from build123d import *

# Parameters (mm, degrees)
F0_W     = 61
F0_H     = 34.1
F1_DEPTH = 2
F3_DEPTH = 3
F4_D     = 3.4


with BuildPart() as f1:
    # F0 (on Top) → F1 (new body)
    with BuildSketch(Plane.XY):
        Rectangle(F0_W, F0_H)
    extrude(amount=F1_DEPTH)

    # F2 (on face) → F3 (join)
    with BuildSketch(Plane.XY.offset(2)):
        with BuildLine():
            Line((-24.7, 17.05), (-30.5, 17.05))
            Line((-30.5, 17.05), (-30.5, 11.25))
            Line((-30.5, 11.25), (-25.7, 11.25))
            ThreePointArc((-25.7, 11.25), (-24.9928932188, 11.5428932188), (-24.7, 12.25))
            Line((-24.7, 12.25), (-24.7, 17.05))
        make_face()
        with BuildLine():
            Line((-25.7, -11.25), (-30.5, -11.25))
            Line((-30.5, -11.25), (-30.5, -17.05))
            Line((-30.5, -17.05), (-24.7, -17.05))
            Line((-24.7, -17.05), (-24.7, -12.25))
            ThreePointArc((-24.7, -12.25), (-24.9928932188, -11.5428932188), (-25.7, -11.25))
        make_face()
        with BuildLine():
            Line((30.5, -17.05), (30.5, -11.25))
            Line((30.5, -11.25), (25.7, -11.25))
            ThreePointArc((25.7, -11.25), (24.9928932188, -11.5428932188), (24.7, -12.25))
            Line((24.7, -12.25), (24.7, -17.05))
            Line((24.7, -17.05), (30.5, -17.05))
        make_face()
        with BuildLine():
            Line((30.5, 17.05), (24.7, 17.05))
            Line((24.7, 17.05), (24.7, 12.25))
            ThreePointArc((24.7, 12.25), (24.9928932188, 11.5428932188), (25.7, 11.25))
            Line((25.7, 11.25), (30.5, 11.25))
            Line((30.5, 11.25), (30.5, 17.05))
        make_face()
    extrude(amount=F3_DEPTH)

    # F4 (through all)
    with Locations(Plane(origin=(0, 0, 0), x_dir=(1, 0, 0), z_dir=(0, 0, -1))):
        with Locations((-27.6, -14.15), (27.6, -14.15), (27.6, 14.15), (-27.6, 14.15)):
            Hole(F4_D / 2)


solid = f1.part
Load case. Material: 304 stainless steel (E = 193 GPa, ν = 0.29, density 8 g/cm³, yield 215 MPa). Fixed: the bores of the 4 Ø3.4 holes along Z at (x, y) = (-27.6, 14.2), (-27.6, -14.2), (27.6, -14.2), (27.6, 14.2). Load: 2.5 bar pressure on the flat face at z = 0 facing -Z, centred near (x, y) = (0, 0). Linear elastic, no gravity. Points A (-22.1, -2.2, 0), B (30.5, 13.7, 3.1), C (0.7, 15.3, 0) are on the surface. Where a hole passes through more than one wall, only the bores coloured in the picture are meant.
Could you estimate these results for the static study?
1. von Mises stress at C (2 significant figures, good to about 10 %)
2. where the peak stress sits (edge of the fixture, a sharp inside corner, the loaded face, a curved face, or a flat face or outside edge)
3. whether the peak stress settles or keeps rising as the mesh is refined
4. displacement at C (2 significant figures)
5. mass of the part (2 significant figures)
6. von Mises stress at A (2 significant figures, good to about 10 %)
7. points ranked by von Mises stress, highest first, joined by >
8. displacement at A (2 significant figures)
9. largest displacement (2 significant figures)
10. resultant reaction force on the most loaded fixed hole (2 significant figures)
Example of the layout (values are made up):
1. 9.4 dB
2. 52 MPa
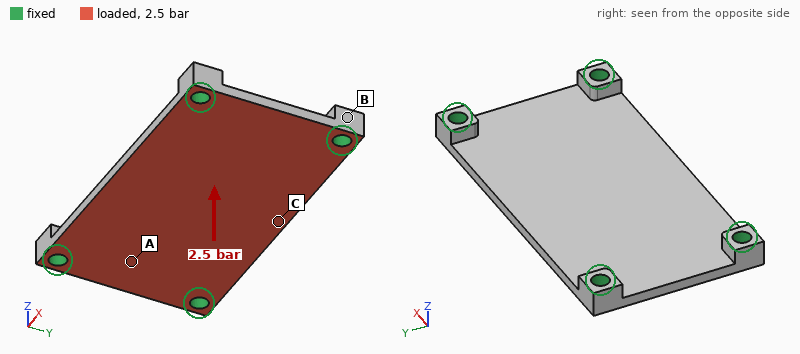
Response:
1. 51 MPa
2. a sharp inside corner
3. keeps rising
4. 46 µm
5. 35 g
6. 28 MPa
7. C > A > B
8. 11 µm
9. 47 µm
10. 130 N
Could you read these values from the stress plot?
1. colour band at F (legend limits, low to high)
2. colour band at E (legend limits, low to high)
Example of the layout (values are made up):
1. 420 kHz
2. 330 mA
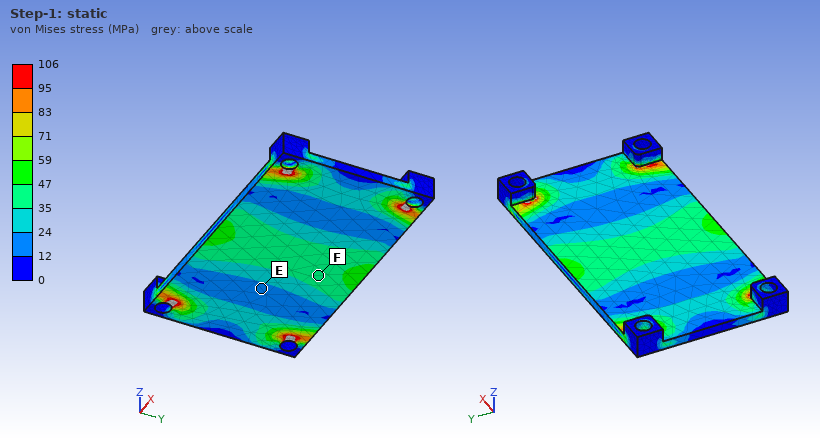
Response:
1. 35 to 47 MPa
2. 12 to 24 MPa
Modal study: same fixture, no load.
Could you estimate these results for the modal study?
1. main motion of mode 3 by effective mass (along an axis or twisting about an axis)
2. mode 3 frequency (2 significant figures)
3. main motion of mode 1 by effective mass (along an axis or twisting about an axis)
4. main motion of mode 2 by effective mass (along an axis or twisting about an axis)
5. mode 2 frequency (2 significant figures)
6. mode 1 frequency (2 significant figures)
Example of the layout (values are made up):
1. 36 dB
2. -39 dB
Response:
1. twisting about Y
2. 8800 Hz
3. along Z
4. twisting about X
5. 5300 Hz
6. 3300 Hz
